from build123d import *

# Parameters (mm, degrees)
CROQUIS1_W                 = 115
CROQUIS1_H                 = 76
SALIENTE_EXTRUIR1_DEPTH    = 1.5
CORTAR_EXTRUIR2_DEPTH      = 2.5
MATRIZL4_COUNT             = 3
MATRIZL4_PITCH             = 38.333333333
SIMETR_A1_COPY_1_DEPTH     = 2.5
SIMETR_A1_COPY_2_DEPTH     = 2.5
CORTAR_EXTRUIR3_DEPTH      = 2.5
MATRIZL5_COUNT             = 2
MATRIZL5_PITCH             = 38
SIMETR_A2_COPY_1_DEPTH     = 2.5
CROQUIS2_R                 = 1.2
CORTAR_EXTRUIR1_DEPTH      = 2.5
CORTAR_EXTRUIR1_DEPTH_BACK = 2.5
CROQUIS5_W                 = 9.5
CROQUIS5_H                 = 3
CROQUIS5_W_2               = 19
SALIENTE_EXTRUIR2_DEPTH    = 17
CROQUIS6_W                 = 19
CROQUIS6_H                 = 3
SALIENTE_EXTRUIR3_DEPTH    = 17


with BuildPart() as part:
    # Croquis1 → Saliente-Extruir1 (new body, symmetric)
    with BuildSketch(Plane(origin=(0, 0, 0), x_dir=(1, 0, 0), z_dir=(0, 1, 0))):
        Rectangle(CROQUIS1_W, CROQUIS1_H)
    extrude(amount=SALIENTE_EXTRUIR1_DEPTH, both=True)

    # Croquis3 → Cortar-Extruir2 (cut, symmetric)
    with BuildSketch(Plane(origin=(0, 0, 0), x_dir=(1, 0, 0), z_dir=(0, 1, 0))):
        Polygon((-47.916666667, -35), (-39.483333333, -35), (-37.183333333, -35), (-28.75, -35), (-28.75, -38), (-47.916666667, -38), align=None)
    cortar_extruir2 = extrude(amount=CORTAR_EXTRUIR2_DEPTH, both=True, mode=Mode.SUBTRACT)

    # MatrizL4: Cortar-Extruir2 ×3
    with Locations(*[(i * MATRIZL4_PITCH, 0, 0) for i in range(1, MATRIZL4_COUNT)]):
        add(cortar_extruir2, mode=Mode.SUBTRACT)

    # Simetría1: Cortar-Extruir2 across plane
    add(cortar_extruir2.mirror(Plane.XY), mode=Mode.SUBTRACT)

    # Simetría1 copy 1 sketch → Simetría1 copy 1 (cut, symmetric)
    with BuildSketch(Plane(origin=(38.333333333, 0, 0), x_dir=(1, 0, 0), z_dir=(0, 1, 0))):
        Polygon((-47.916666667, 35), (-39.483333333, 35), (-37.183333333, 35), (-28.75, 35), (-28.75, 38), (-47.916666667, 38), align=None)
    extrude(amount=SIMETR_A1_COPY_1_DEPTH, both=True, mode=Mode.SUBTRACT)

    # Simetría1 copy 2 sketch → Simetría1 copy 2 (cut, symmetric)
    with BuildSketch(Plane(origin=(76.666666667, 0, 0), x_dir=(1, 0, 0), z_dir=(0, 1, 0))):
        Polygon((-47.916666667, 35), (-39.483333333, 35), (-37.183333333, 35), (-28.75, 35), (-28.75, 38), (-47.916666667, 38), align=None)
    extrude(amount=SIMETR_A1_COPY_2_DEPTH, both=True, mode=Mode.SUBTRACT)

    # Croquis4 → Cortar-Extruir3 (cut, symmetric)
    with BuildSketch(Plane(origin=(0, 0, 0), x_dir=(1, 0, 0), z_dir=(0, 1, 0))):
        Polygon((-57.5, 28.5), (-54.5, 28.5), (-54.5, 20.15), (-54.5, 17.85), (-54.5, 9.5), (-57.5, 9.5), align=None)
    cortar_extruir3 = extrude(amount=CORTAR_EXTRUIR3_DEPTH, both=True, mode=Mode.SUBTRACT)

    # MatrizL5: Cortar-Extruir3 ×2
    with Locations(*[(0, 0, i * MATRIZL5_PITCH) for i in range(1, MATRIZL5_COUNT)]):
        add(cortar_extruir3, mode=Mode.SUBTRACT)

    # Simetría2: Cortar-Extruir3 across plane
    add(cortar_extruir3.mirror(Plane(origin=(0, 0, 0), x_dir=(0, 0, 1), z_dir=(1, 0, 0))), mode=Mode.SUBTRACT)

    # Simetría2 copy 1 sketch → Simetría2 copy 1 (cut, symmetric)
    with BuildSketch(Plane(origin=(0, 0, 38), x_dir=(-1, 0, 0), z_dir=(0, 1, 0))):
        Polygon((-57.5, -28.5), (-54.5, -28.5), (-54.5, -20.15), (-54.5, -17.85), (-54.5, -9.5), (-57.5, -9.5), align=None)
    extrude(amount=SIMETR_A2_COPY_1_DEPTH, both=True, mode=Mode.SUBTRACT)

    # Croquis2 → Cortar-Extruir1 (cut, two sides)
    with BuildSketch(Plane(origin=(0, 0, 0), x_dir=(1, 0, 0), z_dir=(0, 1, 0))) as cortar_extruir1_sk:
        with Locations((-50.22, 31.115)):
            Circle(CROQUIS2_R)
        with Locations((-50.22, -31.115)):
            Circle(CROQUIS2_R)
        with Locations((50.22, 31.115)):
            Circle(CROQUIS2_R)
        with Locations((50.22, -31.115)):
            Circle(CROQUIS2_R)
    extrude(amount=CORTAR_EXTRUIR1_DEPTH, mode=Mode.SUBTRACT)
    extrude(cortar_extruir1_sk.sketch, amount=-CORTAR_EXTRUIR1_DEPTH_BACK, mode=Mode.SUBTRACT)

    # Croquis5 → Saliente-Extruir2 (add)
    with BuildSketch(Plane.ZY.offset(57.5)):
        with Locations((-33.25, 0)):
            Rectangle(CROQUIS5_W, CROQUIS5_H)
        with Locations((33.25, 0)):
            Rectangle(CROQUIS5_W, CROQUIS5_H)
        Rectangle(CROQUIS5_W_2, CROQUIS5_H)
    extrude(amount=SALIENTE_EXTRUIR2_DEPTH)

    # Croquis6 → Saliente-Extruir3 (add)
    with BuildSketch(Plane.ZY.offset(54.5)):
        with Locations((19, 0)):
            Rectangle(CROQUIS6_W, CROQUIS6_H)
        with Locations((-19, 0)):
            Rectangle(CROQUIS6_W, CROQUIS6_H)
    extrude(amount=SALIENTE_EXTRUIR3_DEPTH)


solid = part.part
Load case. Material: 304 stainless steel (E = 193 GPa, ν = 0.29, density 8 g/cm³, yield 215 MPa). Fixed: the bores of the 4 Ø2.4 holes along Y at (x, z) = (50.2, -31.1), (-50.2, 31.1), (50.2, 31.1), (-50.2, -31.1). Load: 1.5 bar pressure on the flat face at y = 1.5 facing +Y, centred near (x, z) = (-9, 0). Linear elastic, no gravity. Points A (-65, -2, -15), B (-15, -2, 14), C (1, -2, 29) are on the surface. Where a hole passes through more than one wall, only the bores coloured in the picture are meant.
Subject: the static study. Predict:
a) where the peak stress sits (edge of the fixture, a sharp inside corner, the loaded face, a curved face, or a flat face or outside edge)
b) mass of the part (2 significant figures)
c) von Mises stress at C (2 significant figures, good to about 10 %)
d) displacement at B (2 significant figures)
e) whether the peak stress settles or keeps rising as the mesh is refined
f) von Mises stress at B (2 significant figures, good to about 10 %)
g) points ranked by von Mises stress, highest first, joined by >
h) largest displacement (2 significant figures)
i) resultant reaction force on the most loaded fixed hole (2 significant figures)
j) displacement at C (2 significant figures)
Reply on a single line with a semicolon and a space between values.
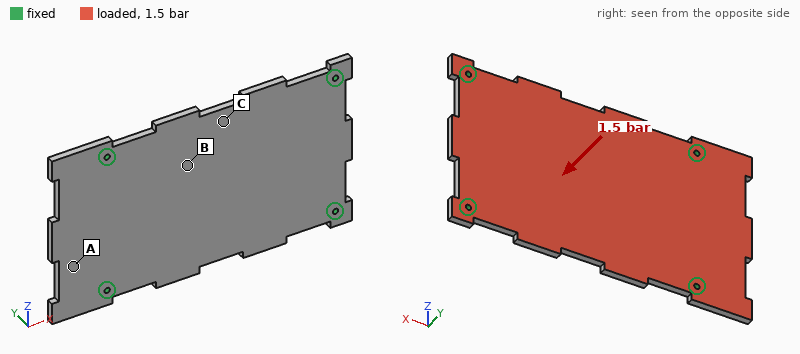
edge of the fixture; 230 g; 59 MPa; 0.13 mm; keeps rising; 37 MPa; C > B > A; 0.15 mm; 410 N; 0.15 mm
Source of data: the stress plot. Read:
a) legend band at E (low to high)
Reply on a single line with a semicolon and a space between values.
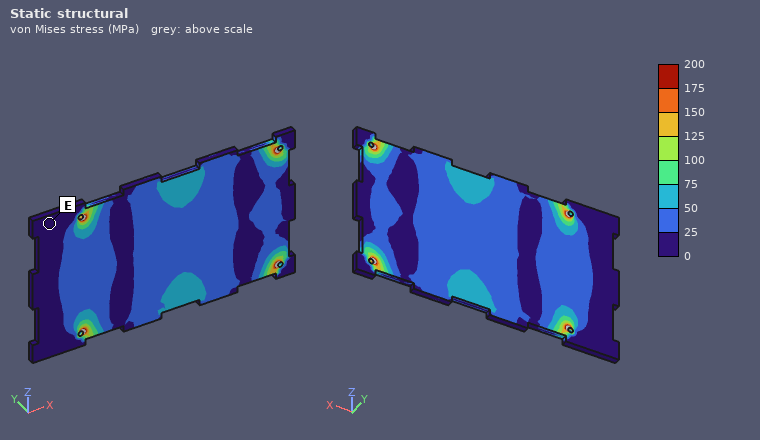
0 to 25 MPa
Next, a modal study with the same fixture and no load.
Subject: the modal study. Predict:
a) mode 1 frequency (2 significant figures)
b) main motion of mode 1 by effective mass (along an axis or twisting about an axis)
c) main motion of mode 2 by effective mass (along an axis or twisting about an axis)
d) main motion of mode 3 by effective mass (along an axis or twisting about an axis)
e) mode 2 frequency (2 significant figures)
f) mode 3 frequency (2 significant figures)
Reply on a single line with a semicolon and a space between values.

1100 Hz; along Y; twisting about X; along Y; 1900 Hz; 2600 Hz
